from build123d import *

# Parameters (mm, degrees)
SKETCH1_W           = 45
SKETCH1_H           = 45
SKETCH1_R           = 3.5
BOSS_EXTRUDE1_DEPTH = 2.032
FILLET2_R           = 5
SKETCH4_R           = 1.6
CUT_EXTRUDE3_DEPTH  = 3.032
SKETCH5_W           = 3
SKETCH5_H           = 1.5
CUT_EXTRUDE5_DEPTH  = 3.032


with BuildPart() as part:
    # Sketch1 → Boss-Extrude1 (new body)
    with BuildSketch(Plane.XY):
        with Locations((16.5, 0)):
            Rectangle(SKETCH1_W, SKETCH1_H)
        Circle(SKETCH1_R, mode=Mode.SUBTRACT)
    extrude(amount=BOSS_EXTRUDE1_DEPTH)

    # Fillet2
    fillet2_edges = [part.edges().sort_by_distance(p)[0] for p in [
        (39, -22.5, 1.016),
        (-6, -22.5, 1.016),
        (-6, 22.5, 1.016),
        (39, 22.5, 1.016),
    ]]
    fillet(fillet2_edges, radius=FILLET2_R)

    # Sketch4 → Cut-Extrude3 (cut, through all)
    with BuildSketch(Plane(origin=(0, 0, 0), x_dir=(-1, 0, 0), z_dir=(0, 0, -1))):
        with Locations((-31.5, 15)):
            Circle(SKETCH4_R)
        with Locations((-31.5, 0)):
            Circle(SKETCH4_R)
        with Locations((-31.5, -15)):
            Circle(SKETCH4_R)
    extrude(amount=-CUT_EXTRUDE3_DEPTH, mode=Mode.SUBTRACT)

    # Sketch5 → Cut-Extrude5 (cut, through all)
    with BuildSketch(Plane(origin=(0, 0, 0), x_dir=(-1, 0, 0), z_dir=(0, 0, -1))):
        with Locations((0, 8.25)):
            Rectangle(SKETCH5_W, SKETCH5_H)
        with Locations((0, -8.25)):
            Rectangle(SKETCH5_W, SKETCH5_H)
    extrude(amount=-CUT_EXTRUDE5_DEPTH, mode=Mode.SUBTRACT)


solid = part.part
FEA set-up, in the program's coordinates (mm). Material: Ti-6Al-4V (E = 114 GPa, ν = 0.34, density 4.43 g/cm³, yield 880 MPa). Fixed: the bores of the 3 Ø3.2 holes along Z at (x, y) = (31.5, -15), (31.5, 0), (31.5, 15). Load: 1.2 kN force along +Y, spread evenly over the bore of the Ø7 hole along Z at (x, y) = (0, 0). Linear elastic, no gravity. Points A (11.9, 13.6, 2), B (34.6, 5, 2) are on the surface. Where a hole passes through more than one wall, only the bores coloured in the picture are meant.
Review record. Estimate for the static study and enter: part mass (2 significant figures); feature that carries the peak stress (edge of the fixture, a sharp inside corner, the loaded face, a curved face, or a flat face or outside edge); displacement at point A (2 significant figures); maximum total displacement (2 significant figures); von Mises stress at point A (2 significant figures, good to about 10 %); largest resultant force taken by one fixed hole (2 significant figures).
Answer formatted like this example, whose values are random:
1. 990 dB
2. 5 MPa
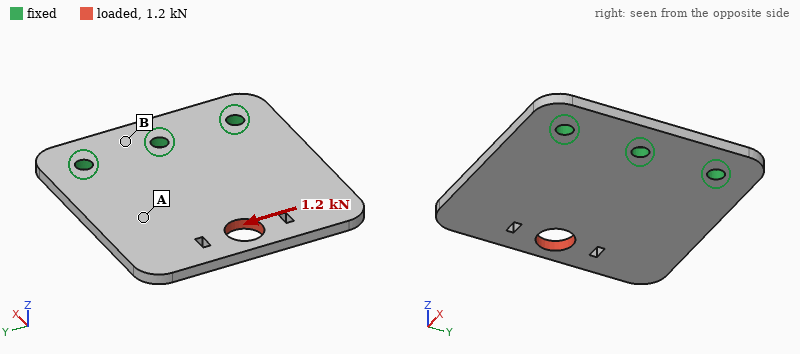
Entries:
1. 17 g
2. edge of the fixture
3. 13 µm
4. 27 µm
5. 24 MPa
6. 1.2 kN
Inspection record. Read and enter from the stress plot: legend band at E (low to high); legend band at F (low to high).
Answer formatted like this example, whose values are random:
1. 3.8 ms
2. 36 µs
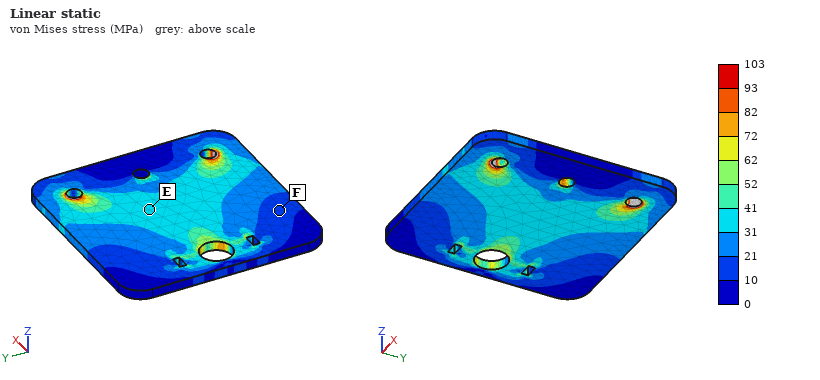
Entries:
1. 31 to 41 MPa
2. 10 to 21 MPa
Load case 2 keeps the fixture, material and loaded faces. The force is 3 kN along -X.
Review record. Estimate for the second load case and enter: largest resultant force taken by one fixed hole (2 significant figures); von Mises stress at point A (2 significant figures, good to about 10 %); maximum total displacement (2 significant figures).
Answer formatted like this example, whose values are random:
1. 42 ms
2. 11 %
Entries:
1. 1.0 kN
2. 32 MPa
3. 28 µm
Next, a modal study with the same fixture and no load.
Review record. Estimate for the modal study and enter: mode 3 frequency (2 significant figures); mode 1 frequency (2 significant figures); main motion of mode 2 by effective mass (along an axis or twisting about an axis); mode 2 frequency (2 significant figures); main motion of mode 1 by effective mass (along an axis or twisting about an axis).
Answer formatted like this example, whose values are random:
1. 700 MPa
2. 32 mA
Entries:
1. 6500 Hz
2. 1300 Hz
3. twisting about X
4. 2600 Hz
5. along Z
